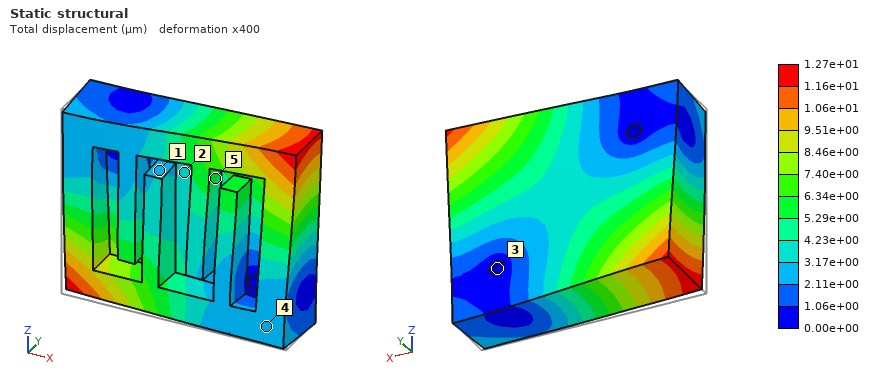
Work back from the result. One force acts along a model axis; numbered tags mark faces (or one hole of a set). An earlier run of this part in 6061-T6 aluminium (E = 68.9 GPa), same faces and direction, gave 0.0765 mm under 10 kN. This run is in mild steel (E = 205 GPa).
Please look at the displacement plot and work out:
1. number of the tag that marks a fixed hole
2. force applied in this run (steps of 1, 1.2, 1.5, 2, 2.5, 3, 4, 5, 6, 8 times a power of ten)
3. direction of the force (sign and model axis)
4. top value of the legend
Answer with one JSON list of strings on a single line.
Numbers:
["3", "5 kN", "+Y", "1.27e+01 µm"]
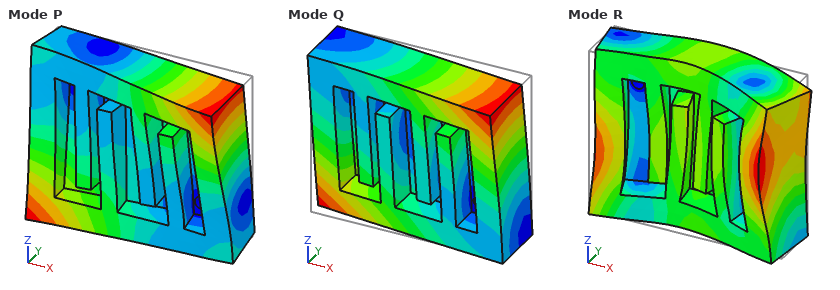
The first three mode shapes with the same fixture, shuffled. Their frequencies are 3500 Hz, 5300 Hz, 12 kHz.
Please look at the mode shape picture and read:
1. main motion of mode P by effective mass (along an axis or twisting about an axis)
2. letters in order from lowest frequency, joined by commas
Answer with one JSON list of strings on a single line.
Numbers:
["along Y", "Q, P, R"]
